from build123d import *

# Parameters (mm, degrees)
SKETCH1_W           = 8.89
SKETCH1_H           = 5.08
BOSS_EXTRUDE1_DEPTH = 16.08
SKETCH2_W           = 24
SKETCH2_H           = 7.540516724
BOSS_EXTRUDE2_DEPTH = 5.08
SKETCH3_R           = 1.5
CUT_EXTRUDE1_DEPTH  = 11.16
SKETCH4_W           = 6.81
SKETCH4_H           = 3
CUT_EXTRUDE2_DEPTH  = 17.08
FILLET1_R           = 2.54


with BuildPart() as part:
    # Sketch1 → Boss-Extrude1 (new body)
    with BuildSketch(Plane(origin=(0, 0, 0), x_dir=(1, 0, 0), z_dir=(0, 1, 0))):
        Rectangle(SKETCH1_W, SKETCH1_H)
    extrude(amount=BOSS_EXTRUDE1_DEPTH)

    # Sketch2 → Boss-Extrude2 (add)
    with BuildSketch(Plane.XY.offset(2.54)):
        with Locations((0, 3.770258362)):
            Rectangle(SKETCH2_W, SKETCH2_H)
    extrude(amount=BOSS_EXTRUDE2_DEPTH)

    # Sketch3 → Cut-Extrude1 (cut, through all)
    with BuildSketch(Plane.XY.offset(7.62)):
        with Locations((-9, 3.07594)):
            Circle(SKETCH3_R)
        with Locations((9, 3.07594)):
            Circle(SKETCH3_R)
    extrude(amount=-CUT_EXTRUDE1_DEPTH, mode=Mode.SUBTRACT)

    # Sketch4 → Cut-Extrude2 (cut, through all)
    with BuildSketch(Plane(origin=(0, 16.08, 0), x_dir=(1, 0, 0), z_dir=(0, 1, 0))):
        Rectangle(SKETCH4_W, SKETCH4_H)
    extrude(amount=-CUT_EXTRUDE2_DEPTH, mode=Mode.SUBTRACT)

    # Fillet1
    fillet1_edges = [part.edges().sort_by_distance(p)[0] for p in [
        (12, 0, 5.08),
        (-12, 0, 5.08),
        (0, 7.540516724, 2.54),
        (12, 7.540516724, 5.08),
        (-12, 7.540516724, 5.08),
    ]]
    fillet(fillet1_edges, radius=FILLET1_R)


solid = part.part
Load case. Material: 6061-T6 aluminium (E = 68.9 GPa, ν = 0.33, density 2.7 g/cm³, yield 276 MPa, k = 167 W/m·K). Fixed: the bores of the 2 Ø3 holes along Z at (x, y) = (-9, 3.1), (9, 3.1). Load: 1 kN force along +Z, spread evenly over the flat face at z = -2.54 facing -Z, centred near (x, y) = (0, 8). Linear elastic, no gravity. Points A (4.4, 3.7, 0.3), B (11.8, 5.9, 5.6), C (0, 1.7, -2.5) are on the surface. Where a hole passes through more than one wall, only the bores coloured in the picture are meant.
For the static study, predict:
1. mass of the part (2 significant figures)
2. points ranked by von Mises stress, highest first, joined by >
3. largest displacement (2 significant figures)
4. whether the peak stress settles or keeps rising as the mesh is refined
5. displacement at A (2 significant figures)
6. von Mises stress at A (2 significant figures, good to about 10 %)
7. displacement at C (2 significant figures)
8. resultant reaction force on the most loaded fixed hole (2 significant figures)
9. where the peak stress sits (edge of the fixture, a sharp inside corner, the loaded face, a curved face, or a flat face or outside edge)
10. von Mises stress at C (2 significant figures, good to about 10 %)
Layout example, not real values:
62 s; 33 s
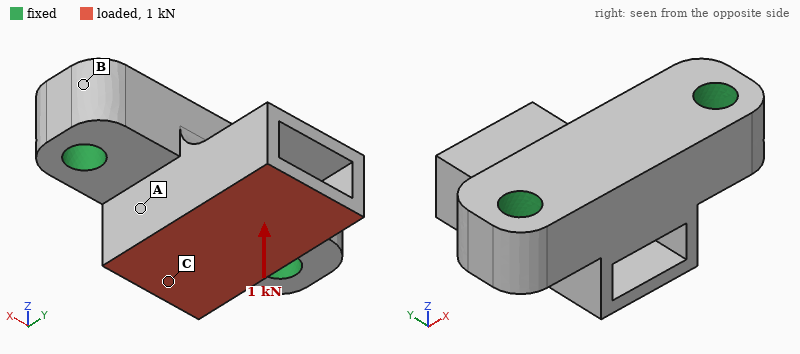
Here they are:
3.3 g; C > A > B; 96 µm; keeps rising; 15 µm; 66 MPa; 31 µm; 510 N; a sharp inside corner; 130 MPa
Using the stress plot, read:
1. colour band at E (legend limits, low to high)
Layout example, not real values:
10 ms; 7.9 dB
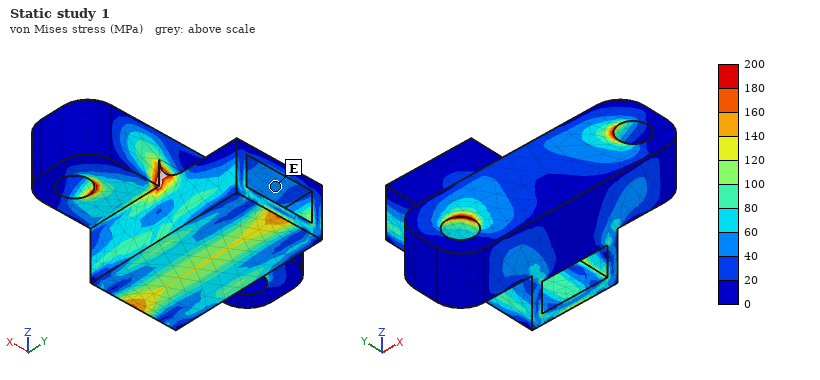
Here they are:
40 to 60 MPa
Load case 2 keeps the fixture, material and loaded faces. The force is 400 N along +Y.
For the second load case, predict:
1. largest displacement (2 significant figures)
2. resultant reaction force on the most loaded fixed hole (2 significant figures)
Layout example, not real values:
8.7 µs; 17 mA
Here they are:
43 µm; 200 N
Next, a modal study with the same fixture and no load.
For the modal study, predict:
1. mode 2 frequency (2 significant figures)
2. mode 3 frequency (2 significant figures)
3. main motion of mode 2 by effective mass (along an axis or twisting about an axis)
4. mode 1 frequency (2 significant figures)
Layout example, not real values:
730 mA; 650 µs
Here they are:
27 kHz; 35 kHz; along X; 19 kHz
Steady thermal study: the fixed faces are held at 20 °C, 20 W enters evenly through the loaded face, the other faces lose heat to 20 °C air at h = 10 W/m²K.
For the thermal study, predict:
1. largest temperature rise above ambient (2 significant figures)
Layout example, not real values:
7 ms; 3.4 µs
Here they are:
42 K
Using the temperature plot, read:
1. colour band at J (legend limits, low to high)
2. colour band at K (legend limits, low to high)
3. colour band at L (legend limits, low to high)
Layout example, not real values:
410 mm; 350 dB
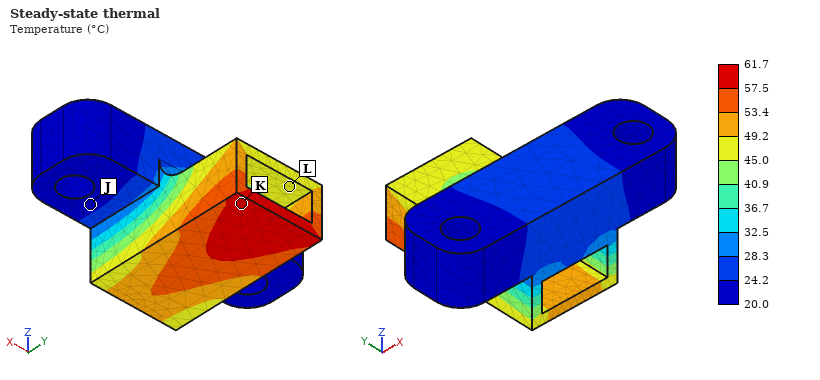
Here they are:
20.0 to 24.2 °C; 57.5 to 61.7 °C; 45.0 to 49.2 °C
